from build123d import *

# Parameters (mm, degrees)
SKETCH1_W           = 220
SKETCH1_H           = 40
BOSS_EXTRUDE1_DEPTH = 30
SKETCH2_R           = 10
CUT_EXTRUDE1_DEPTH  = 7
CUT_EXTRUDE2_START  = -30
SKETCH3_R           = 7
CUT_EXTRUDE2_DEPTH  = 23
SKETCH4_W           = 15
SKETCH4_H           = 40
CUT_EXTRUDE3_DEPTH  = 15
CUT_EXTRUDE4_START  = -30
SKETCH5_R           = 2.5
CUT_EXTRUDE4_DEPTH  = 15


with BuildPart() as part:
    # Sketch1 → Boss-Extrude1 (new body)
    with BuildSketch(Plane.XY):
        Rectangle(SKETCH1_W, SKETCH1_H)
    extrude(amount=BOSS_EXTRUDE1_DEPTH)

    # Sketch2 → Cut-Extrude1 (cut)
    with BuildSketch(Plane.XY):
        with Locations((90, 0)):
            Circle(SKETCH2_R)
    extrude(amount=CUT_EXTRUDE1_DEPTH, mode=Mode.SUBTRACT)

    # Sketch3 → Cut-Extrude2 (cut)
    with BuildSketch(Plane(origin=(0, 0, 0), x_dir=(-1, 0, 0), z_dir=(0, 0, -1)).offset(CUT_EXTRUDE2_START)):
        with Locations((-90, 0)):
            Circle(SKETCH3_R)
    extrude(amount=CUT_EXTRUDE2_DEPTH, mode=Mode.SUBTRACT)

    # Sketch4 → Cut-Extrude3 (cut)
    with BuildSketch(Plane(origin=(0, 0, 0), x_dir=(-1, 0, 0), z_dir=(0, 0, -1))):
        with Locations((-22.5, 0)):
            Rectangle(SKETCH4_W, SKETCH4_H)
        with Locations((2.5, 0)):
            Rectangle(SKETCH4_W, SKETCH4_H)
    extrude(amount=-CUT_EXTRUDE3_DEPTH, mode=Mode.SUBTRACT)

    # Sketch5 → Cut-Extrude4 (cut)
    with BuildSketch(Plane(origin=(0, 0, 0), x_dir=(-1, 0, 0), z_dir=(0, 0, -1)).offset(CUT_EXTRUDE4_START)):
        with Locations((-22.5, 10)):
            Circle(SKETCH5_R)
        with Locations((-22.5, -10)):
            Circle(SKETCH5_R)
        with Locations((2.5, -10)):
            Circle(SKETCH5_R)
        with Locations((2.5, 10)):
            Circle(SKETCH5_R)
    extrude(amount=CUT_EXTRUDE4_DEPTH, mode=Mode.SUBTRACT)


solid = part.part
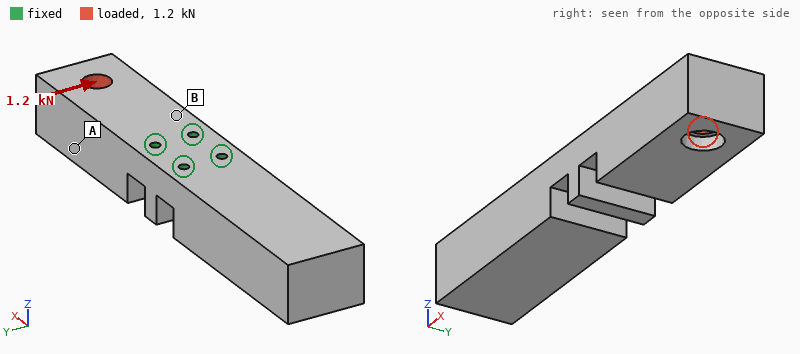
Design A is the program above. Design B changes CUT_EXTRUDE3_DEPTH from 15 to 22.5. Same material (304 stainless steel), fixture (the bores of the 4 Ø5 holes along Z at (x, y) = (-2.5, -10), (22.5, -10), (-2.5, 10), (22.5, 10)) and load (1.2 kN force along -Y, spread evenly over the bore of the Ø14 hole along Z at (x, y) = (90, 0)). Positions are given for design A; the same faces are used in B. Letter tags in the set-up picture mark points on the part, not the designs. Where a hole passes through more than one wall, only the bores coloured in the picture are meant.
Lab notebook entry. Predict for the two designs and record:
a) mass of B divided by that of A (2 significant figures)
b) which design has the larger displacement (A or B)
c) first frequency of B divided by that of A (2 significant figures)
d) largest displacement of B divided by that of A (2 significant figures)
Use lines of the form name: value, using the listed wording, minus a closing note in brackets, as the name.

mass of B divided by that of A: 0.96
which design has the larger displacement: B
first frequency of B divided by that of A: 0.43
largest displacement of B divided by that of A: 1.7
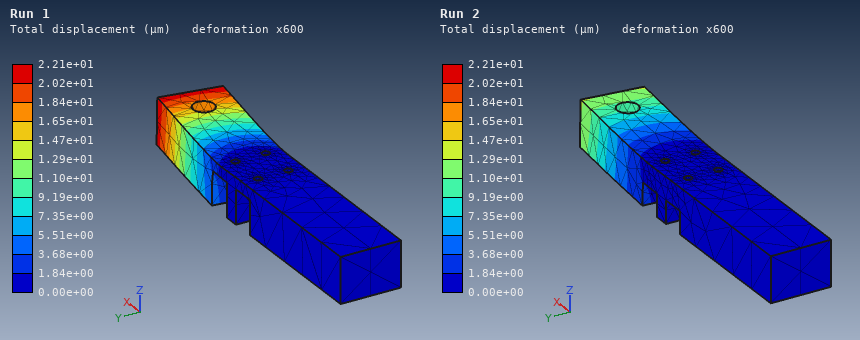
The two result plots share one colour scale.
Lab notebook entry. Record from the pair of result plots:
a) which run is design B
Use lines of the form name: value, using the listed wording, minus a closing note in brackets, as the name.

which run is design B: Run 1
